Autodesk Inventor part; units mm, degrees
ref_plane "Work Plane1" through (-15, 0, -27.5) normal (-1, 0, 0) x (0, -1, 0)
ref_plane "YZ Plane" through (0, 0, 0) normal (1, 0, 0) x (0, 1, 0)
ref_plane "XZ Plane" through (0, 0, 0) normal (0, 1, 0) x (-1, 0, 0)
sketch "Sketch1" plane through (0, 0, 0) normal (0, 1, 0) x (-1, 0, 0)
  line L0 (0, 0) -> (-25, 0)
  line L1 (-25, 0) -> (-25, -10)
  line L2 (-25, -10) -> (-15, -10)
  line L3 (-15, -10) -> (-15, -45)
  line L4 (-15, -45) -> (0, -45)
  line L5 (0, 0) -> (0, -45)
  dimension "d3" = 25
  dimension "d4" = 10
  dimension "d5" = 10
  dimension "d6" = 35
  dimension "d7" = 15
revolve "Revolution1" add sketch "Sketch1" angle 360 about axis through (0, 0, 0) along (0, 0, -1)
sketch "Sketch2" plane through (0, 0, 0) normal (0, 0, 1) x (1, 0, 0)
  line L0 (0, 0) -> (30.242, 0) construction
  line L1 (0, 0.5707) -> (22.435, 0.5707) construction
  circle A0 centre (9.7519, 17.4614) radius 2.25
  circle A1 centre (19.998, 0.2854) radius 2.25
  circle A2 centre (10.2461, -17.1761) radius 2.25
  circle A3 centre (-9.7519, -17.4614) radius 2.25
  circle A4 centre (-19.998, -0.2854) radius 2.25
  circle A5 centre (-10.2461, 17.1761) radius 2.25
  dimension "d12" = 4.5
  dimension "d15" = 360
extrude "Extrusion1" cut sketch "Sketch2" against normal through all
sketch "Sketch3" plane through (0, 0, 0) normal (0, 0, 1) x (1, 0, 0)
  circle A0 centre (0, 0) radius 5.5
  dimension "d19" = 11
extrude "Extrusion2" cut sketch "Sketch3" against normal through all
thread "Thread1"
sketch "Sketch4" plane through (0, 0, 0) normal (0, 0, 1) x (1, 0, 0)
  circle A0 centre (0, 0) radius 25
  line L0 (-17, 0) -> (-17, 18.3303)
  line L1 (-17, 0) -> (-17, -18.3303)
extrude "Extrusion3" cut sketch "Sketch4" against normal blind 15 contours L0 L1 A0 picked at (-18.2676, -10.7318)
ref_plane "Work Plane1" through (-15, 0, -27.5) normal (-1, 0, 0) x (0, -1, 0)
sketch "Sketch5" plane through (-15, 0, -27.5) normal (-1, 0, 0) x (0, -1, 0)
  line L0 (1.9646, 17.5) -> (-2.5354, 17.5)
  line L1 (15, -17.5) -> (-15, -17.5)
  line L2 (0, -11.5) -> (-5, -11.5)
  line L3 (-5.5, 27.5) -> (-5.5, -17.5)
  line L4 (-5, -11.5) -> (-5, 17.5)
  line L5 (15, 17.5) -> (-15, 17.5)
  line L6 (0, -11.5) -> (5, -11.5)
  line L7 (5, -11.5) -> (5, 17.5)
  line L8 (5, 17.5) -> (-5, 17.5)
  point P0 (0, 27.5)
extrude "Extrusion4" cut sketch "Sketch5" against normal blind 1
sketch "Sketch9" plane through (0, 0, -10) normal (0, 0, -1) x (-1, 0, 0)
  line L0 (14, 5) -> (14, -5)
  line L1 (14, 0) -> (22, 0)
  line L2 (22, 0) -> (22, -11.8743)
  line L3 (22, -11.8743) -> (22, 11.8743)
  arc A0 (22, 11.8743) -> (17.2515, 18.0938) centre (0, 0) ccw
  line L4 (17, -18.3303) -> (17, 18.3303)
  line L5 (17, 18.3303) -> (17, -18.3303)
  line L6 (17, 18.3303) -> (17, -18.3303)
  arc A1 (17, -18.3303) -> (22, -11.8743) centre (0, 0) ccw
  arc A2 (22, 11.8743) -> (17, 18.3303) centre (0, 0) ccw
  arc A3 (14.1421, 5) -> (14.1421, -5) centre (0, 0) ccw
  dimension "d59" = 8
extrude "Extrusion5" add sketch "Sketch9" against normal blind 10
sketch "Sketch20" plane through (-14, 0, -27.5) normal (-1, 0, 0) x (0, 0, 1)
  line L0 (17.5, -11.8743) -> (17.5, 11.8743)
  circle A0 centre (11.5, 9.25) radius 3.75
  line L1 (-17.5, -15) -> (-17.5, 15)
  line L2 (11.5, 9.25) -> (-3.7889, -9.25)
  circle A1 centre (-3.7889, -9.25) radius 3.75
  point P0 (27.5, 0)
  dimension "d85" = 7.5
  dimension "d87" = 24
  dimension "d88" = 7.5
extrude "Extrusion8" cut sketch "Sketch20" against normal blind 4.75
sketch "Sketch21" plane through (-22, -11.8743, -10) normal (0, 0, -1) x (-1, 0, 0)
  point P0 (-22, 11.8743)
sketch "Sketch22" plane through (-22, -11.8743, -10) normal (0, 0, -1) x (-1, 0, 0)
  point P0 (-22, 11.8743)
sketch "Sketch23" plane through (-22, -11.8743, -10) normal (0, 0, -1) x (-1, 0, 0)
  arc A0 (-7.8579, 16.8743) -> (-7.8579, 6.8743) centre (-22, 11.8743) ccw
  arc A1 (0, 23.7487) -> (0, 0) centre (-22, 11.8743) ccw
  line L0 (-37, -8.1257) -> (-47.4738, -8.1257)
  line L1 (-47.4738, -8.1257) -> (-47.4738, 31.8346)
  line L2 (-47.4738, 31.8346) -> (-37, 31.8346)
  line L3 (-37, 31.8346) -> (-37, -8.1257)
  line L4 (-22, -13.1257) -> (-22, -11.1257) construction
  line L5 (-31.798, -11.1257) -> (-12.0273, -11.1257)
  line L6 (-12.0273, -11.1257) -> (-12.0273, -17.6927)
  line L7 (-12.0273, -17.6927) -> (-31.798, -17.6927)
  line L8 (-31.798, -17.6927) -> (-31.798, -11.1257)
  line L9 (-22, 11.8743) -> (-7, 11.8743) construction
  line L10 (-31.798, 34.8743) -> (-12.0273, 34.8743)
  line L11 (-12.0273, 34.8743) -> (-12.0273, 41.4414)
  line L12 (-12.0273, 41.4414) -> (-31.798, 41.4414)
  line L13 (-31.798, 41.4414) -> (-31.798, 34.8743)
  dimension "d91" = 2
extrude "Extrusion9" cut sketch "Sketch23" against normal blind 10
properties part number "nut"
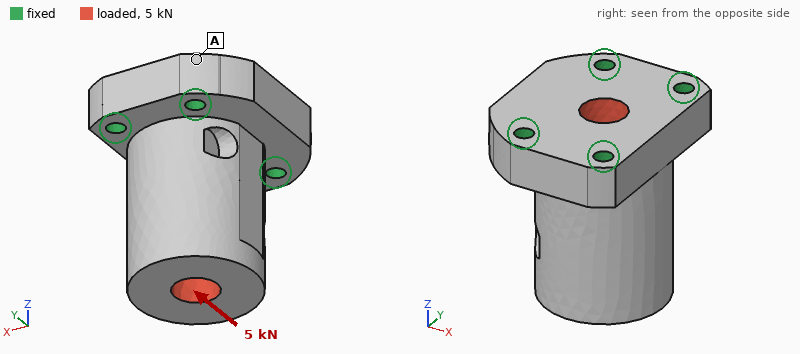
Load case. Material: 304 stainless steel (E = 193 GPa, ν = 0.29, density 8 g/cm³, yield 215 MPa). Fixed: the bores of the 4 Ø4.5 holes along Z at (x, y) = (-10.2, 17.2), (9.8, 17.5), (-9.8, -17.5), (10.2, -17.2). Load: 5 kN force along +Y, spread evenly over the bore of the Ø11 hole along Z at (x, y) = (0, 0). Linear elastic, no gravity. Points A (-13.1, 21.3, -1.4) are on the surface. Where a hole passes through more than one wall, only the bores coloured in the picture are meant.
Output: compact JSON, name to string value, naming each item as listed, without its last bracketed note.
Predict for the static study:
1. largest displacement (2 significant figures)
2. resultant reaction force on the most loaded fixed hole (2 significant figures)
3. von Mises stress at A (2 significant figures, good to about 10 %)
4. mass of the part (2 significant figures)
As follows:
{"largest displacement": "9.2 µm", "resultant reaction force on the most loaded fixed hole": "1.9 kN", "von Mises stress at A": "7.8 MPa", "mass of the part": "280 g"}
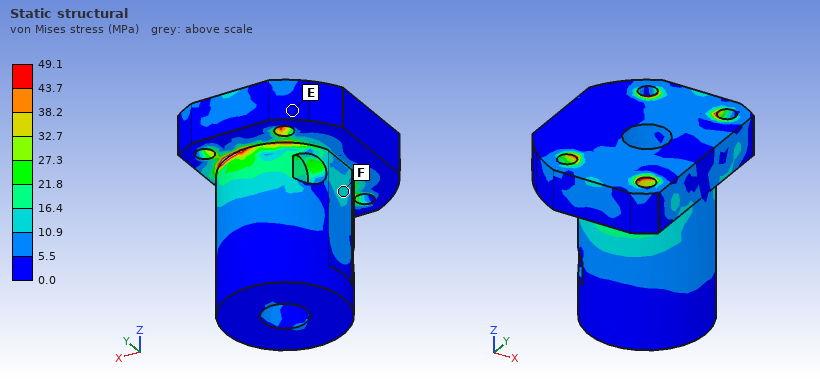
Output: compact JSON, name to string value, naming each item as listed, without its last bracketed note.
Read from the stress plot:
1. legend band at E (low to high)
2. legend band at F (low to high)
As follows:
{"legend band at E": "0.0 to 5.5 MPa", "legend band at F": "10.9 to 16.4 MPa"}
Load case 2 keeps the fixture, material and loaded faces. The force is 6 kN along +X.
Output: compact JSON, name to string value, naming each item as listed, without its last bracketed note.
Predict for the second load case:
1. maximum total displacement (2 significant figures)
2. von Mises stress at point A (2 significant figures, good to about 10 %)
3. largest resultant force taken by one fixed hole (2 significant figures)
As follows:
{"maximum total displacement": "19 µm", "von Mises stress at point A": "17 MPa", "largest resultant force taken by one fixed hole": "2.8 kN"}
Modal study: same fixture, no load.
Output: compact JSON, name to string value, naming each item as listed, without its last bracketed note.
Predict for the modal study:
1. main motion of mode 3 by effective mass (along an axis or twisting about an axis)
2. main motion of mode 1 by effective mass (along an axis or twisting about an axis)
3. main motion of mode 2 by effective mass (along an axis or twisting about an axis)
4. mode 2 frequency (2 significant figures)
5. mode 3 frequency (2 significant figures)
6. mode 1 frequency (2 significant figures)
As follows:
{"main motion of mode 3 by effective mass": "along Z", "main motion of mode 1 by effective mass": "along X", "main motion of mode 2 by effective mass": "along Y", "mode 2 frequency": "9500 Hz", "mode 3 frequency": "18 kHz", "mode 1 frequency": "7200 Hz"}
